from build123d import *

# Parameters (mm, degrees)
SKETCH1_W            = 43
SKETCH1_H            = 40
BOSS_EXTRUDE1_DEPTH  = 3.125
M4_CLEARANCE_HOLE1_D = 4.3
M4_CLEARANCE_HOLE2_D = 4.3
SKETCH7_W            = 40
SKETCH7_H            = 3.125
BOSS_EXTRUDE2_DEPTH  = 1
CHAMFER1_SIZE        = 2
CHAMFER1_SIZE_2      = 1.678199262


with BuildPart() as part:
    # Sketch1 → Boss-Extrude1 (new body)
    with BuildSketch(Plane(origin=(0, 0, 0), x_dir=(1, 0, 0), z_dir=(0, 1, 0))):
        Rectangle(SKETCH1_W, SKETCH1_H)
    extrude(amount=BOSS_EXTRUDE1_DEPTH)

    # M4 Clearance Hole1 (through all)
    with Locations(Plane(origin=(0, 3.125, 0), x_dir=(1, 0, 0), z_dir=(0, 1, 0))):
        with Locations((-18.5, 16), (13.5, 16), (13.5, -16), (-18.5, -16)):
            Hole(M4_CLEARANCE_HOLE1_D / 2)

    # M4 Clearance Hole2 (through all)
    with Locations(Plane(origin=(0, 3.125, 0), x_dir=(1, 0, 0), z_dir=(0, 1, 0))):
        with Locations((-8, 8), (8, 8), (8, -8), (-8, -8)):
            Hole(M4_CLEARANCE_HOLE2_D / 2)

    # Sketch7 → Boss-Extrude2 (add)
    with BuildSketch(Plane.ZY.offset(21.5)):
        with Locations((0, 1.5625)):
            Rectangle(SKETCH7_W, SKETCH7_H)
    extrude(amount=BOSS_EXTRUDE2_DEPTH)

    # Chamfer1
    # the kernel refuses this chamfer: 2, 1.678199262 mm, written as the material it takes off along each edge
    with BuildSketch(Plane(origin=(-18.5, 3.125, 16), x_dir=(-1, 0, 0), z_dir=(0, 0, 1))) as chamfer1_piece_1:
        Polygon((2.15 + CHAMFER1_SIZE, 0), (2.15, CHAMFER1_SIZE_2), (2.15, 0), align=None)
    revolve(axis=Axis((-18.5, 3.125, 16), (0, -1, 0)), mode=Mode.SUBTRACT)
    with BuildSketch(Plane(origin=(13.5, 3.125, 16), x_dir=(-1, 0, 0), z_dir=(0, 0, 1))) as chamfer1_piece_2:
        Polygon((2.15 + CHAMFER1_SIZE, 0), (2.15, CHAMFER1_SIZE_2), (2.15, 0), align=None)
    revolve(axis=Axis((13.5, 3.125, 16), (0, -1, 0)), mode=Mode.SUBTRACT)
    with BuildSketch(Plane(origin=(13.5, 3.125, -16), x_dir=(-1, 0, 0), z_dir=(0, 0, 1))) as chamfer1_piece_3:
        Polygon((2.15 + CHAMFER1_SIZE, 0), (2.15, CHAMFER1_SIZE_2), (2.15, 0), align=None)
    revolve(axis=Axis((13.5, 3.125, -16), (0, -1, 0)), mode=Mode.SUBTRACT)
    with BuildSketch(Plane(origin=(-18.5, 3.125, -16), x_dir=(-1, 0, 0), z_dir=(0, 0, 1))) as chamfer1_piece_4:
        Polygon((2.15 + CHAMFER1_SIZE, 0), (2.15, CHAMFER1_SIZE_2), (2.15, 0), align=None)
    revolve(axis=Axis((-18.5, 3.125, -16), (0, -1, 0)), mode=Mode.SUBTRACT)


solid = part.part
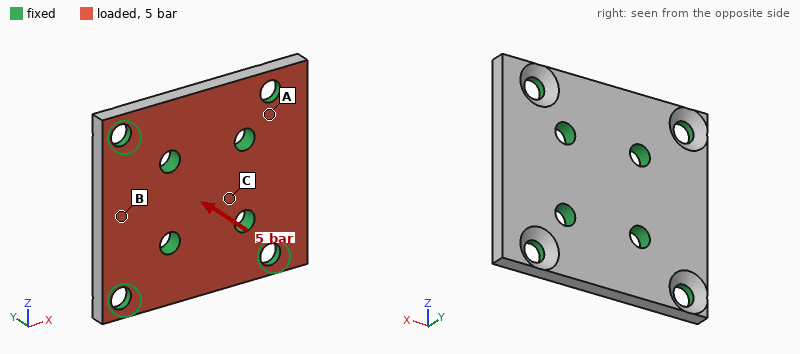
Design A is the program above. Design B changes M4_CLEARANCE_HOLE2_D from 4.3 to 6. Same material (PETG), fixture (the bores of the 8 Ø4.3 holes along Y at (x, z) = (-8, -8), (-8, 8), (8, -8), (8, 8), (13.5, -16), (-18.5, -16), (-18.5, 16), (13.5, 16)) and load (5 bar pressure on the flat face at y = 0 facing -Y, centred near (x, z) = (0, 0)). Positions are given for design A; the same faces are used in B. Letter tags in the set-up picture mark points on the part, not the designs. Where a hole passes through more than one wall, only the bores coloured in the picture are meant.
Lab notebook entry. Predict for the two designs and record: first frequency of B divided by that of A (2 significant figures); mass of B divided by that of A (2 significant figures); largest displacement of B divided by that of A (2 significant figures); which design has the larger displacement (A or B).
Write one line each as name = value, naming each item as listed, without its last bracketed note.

first frequency of B divided by that of A = 1.1
mass of B divided by that of A = 0.97
largest displacement of B divided by that of A = 0.83
which design has the larger displacement = A
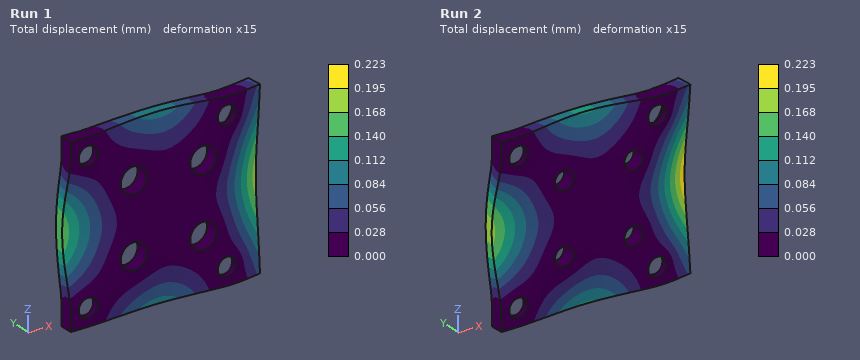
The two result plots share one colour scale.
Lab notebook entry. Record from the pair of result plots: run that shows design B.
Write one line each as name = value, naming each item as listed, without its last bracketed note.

run that shows design B = Run 1
